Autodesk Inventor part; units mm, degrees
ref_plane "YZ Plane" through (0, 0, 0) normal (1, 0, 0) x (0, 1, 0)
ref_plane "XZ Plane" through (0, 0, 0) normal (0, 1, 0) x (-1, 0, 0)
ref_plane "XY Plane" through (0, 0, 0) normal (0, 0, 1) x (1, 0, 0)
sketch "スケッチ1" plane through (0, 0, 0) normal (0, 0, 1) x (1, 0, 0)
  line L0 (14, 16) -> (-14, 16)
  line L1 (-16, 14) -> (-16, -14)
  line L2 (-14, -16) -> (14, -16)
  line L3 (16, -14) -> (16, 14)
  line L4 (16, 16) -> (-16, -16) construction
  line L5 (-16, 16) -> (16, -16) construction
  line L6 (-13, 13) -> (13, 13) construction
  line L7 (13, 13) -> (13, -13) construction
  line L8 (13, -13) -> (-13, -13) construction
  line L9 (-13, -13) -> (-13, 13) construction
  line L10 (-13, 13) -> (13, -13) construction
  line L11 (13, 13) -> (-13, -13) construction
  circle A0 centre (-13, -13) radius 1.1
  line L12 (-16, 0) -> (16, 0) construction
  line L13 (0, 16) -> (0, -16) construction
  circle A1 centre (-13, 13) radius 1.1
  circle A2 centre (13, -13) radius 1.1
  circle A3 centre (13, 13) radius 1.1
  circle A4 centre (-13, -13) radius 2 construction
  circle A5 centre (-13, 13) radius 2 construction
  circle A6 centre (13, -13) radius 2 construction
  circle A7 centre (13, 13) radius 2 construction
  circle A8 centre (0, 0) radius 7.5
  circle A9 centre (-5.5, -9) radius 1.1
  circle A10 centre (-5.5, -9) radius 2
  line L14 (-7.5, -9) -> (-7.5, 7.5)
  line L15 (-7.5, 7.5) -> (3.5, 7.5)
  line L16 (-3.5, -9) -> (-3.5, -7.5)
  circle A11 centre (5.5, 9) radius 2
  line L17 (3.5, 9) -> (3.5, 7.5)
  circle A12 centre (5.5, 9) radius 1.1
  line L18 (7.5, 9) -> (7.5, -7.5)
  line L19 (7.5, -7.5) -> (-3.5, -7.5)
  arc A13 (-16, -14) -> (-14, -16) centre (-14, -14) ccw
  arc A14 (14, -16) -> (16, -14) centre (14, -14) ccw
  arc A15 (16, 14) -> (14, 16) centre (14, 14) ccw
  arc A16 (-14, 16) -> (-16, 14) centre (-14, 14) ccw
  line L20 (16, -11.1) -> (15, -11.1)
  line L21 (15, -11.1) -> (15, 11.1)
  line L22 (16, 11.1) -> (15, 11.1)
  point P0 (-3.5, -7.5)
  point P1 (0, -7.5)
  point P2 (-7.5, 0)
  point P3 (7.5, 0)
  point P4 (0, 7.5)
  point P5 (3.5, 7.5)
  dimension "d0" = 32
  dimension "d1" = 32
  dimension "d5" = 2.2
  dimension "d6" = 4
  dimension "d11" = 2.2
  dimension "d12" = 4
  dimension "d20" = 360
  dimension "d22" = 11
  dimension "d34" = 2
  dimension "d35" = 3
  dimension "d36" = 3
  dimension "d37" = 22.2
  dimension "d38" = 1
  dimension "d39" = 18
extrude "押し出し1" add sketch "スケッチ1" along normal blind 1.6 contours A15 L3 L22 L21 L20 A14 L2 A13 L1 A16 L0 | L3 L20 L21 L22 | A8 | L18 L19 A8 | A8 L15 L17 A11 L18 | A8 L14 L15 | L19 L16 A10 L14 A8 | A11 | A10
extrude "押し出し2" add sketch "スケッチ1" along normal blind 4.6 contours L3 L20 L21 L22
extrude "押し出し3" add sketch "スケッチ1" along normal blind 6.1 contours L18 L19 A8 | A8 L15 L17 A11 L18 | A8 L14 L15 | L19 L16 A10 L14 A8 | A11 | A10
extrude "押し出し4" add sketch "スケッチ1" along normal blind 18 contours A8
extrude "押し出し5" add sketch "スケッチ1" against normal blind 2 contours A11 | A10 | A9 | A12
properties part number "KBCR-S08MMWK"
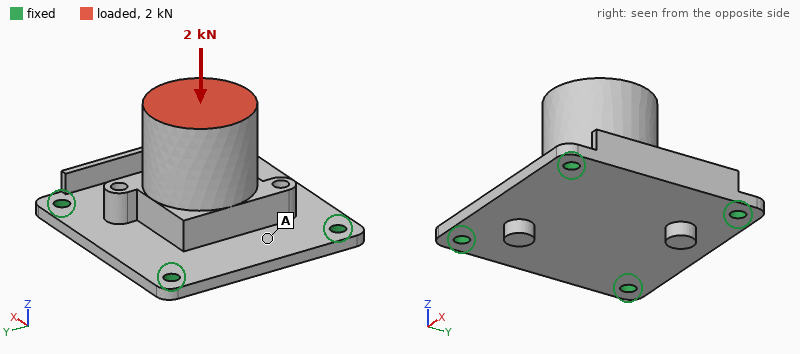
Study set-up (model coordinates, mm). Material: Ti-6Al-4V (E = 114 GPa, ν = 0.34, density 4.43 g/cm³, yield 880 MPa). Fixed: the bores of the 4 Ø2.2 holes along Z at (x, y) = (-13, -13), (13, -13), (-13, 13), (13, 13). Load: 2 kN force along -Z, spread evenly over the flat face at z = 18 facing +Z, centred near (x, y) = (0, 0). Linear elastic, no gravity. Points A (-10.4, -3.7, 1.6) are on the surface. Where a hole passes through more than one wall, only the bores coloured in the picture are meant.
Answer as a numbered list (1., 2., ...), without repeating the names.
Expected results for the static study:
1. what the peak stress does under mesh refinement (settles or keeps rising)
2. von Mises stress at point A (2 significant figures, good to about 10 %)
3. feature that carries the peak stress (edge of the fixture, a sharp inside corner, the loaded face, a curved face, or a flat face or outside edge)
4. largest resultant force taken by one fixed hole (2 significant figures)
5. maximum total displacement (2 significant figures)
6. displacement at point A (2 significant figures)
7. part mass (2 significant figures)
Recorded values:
1. keeps rising
2. 100 MPa
3. edge of the fixture
4. 660 N
5. 75 µm
6. 61 µm
7. 22 g
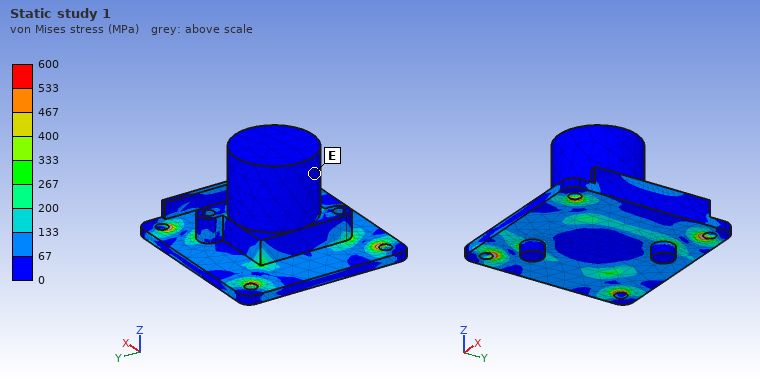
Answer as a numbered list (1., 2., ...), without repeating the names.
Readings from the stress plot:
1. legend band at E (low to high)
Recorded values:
1. 0 to 67 MPa
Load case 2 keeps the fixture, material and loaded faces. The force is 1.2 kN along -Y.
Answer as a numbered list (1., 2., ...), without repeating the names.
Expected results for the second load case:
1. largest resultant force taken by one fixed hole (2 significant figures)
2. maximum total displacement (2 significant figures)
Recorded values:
1. 580 N
2. 0.13 mm
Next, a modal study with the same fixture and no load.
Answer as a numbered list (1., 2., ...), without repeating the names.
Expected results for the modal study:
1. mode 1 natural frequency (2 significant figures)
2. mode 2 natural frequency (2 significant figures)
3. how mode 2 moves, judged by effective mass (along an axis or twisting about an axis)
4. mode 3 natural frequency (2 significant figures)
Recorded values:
1. 6000 Hz
2. 6300 Hz
3. along Z
4. 7200 Hz
